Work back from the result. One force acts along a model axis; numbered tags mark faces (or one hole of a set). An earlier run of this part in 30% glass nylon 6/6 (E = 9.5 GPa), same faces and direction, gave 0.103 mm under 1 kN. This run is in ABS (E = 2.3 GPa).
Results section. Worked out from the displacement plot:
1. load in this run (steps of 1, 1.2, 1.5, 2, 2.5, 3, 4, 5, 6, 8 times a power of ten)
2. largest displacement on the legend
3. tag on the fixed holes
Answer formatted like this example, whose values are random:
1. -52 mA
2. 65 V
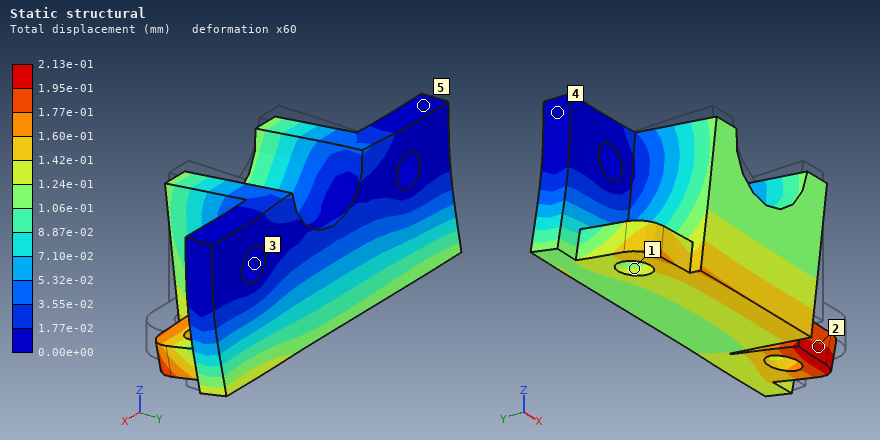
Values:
1. 500 N
2. 2.13e-01 mm
3. 3
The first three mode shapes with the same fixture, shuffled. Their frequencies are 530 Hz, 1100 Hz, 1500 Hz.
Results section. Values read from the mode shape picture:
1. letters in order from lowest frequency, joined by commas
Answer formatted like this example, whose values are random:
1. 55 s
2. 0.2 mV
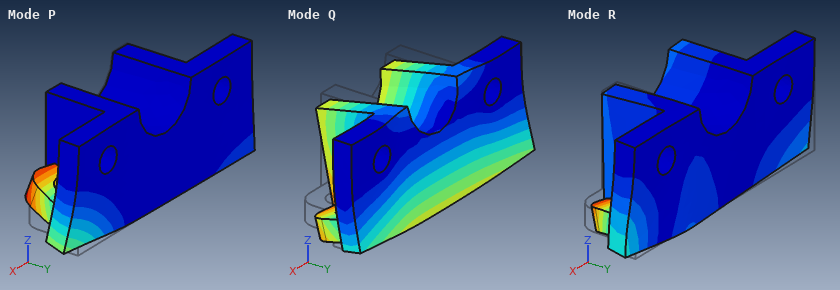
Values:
1. Q, P, R
